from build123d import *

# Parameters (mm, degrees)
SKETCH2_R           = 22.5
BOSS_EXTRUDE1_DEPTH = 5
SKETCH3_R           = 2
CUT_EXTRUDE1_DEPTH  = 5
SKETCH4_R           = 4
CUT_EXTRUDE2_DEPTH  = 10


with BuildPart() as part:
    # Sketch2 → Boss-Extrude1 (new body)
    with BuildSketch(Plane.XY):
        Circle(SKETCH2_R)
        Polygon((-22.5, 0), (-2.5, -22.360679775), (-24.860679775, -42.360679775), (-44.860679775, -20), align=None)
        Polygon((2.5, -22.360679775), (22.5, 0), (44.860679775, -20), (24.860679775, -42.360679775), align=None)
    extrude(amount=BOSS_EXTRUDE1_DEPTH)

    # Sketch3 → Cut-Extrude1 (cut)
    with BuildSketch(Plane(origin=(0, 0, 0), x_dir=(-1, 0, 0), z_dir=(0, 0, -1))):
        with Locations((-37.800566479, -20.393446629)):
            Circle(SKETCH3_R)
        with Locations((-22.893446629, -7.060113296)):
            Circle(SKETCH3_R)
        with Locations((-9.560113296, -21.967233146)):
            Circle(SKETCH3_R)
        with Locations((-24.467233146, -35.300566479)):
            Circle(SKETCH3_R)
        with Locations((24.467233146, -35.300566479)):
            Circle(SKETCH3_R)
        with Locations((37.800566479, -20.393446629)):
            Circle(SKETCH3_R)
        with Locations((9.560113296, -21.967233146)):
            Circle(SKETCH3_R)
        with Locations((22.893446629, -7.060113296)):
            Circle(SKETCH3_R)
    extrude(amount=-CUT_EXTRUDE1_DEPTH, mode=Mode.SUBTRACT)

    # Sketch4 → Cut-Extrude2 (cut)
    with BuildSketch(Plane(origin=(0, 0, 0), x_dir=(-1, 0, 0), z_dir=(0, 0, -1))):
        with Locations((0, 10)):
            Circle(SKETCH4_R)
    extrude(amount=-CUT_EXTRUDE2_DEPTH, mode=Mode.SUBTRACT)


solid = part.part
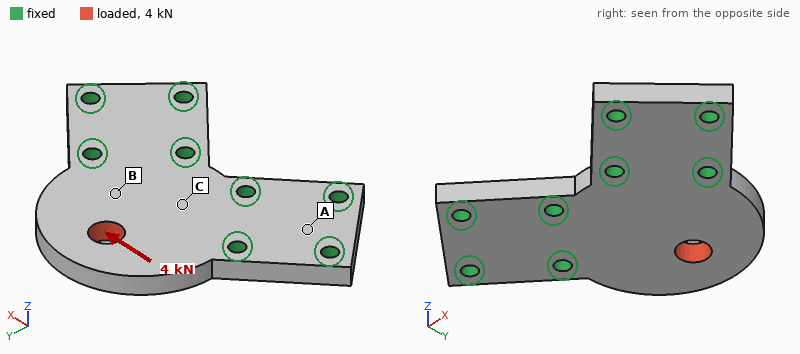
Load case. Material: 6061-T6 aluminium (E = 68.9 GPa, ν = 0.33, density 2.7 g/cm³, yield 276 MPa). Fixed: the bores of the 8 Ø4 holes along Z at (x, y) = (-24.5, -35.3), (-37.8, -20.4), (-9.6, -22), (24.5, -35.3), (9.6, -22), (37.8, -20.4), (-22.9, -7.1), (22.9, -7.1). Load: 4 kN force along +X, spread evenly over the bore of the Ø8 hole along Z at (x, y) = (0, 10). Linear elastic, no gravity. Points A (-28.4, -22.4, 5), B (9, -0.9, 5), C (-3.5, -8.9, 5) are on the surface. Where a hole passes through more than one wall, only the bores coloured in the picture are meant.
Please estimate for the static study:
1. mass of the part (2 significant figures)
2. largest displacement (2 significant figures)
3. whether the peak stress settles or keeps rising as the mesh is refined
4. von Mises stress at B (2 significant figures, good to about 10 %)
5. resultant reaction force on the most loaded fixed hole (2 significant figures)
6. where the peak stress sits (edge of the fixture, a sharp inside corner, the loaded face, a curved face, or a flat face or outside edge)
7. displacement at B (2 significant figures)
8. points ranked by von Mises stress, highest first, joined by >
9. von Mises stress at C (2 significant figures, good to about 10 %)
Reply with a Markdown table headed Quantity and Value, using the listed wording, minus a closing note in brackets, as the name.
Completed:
| Quantity | Value |
|---|---|
| mass of the part | 41 g |
| largest displacement | 22 µm |
| whether the peak stress settles or keeps rising as the mesh is refined | keeps rising |
| von Mises stress at B | 28 MPa |
| resultant reaction force on the most loaded fixed hole | 2.1 kN |
| where the peak stress sits | edge of the fixture |
| displacement at B | 6.2 µm |
| points ranked by von Mises stress, highest first, joined by > | B > C > A |
| von Mises stress at C | 14 MPa |
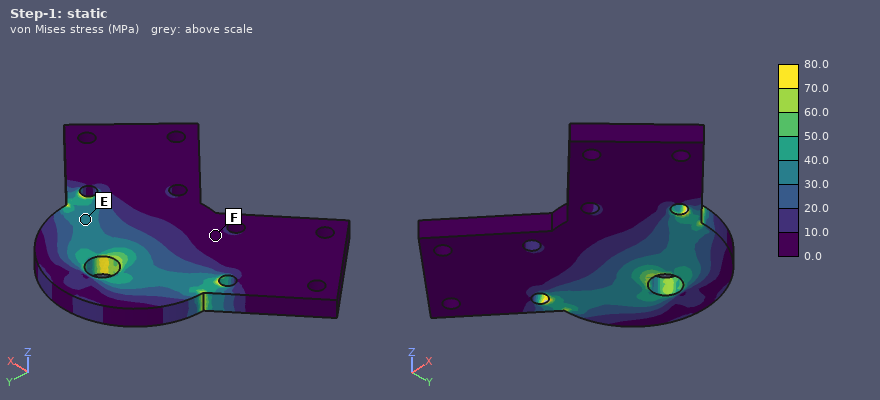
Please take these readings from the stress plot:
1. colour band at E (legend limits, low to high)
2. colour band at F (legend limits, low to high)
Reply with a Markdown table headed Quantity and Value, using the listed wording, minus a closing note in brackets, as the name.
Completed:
| Quantity | Value |
|---|---|
| colour band at E | 30.0 to 40.0 MPa |
| colour band at F | 0.0 to 10.0 MPa |
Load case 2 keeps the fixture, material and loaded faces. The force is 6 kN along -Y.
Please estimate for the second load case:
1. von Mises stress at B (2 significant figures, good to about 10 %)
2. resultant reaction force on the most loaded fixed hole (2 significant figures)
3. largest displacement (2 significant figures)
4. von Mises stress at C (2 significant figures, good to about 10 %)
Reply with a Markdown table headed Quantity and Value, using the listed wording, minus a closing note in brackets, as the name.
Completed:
| Quantity | Value |
|---|---|
| von Mises stress at B | 31 MPa |
| resultant reaction force on the most loaded fixed hole | 1.6 kN |
| largest displacement | 21 µm |
| von Mises stress at C | 26 MPa |
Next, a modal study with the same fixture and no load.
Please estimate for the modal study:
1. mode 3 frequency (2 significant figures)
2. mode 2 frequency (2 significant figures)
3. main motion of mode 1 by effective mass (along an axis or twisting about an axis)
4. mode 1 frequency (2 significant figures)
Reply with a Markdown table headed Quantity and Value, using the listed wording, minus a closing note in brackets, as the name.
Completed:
| Quantity | Value |
|---|---|
| mode 3 frequency | 18 kHz |
| mode 2 frequency | 12 kHz |
| main motion of mode 1 by effective mass | along Z |
| mode 1 frequency | 4700 Hz |
